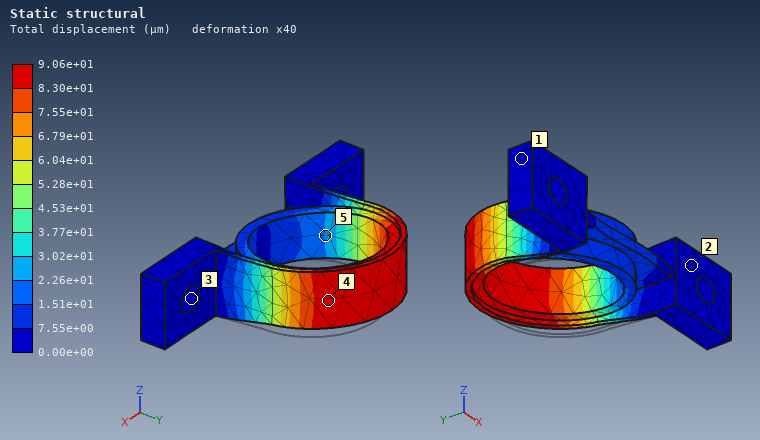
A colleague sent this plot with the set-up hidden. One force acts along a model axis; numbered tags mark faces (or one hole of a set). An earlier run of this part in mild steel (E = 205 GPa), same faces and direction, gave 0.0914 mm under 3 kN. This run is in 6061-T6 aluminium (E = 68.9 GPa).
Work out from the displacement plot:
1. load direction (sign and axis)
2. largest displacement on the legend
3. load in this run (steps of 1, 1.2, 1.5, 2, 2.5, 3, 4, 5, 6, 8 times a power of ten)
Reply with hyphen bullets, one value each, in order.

- -X
- 9.06e+01 µm
- 1 kN
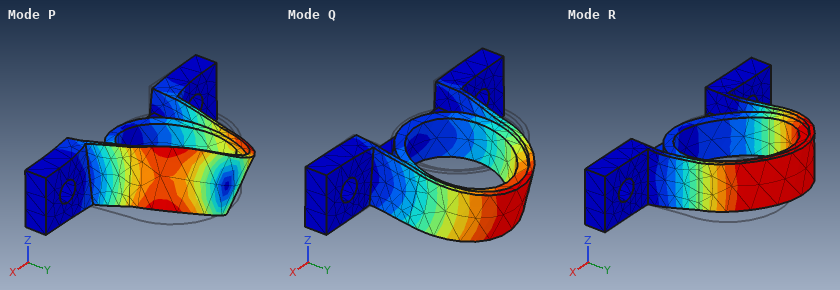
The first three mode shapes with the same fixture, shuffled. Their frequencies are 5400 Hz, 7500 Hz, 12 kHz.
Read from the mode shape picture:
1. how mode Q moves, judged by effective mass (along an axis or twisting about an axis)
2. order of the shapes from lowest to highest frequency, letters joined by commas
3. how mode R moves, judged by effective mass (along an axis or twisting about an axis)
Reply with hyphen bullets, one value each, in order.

- along Z
- Q, R, P
- along X
